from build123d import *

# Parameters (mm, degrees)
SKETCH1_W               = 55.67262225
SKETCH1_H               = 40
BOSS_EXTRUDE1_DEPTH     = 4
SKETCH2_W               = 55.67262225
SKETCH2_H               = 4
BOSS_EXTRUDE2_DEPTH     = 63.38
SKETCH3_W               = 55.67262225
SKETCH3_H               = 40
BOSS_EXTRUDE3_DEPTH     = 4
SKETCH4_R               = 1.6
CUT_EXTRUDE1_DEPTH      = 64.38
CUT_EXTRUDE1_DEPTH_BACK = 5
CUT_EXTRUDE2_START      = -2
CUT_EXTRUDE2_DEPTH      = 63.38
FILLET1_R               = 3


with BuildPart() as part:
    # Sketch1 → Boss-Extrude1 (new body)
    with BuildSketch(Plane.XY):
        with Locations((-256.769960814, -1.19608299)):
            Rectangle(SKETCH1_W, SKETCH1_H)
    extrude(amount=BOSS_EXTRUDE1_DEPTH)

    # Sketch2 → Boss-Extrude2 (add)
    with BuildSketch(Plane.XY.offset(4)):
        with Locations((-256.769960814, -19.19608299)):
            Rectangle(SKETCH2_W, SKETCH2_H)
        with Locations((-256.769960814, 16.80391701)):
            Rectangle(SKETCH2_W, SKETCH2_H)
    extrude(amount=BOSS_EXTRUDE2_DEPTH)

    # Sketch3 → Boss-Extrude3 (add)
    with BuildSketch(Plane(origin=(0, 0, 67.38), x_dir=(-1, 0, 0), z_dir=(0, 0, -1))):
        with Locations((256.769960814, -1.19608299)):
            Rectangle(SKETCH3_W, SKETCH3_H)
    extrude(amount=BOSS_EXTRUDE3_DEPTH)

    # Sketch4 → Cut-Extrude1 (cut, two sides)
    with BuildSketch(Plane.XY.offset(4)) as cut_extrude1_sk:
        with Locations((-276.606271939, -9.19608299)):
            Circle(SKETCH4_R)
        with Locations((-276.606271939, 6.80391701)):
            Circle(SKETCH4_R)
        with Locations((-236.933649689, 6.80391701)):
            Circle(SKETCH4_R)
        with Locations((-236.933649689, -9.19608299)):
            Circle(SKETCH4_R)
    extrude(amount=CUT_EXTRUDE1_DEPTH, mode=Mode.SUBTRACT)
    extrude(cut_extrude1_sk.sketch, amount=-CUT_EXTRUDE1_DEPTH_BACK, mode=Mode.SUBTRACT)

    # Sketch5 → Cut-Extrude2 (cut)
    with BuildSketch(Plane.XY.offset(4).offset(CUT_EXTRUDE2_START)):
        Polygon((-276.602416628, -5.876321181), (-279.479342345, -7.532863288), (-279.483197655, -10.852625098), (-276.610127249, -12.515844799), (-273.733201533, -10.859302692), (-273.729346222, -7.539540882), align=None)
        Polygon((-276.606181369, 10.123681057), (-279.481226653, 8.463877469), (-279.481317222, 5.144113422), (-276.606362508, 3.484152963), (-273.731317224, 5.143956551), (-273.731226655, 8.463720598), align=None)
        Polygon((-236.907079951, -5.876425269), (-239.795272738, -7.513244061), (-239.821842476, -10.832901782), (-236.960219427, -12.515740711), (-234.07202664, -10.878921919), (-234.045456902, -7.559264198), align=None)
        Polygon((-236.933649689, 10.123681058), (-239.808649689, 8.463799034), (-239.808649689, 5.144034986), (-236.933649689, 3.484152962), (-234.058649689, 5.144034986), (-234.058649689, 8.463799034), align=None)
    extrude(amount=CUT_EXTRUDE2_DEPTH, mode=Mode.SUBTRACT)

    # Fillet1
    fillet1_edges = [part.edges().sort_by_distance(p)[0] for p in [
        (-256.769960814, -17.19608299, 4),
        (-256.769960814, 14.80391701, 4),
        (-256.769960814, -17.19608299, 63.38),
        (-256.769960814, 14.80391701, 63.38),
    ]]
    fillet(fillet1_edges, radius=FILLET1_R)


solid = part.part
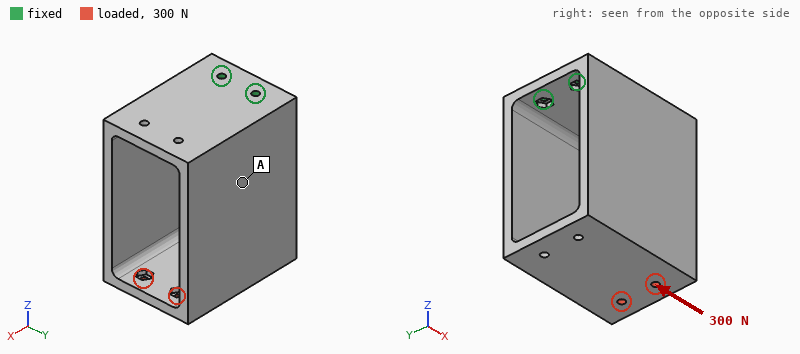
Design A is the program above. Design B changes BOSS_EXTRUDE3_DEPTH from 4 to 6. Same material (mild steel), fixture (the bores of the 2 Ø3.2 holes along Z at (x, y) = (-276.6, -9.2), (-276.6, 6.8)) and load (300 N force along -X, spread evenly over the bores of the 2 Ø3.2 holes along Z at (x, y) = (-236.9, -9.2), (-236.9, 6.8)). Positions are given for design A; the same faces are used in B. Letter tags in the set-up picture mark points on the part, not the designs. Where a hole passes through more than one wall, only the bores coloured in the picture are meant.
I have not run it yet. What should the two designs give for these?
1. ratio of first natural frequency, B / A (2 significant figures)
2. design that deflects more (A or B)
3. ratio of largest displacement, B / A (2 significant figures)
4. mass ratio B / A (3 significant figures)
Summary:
1.1
A
0.78
1.08
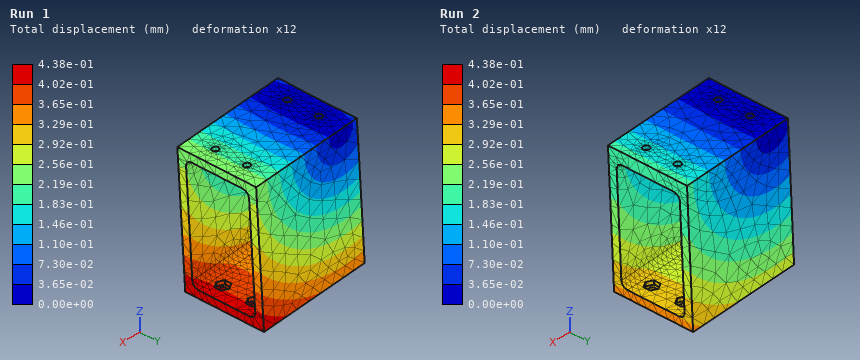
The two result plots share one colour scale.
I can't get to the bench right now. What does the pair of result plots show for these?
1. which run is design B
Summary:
Run 2
